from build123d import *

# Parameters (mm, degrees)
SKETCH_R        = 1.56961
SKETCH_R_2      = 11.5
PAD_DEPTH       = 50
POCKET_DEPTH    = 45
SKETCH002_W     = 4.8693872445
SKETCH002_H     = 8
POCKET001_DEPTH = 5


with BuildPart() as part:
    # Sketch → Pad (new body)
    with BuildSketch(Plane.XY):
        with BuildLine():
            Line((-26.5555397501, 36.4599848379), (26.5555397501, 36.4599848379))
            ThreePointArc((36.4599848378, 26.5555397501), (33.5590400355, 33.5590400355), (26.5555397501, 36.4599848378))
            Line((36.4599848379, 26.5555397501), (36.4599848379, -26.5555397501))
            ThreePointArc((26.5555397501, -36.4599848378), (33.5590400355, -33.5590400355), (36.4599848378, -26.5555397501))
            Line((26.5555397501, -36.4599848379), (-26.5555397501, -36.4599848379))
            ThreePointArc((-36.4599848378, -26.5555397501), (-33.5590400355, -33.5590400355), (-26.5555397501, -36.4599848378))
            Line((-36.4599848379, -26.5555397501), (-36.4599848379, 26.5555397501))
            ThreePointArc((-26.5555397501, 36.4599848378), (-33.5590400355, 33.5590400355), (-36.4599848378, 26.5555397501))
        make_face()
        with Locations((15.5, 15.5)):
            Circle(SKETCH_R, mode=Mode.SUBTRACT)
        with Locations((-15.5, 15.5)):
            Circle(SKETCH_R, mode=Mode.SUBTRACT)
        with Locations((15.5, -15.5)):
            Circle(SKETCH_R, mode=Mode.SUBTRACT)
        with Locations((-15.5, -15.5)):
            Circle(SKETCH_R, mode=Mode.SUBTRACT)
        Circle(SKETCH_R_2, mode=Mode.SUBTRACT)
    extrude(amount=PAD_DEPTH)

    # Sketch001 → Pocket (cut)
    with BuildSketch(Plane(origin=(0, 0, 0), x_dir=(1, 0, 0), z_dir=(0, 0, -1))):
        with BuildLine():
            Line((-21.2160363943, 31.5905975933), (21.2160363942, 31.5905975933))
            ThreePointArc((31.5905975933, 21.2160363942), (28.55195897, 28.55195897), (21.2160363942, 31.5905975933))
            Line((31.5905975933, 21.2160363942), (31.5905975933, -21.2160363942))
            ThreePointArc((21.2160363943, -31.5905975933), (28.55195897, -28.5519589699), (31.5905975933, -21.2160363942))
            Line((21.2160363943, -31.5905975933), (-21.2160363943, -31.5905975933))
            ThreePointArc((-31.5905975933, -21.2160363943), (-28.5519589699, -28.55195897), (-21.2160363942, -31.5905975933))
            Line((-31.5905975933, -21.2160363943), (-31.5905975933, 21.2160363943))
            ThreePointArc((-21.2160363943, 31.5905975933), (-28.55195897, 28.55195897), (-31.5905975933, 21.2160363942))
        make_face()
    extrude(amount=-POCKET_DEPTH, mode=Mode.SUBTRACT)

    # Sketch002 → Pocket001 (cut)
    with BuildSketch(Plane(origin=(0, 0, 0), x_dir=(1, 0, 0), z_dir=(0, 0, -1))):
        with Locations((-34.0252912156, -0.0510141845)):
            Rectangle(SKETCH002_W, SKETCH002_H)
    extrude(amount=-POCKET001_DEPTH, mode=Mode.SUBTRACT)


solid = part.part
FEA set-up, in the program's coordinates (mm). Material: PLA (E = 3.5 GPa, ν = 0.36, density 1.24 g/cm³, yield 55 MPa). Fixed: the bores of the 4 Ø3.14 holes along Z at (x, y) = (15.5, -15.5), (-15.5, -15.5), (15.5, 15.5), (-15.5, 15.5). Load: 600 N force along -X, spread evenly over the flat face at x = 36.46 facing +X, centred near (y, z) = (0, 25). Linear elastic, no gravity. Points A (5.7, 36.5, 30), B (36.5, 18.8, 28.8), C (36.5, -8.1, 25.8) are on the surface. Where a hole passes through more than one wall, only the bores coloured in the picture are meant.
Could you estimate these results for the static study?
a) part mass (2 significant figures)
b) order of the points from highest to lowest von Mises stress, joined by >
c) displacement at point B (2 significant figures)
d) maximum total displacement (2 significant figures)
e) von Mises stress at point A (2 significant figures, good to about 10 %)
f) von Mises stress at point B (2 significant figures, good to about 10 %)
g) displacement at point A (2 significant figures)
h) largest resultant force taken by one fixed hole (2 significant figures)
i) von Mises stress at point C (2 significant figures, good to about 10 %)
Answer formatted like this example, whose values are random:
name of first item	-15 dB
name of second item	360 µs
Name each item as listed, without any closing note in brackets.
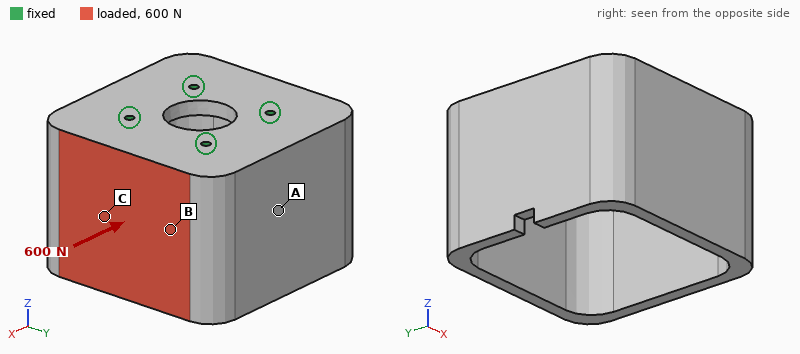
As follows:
part mass	100 g
order of the points from highest to lowest von Mises stress, joined by >	C > B > A
displacement at point B	0.32 mm
maximum total displacement	0.79 mm
von Mises stress at point A	2.2 MPa
von Mises stress at point B	4.7 MPa
displacement at point A	0.13 mm
largest resultant force taken by one fixed hole	300 N
von Mises stress at point C	6.2 MPa
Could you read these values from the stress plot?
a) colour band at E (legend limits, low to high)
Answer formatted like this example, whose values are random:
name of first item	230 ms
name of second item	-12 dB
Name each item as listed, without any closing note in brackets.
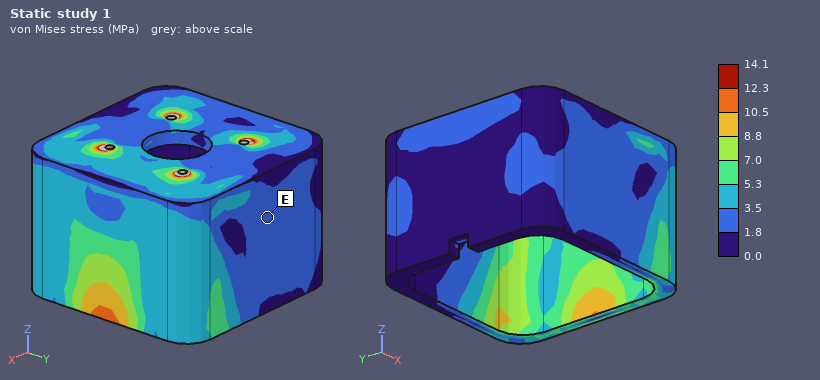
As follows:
colour band at E	1.8 to 3.5 MPa
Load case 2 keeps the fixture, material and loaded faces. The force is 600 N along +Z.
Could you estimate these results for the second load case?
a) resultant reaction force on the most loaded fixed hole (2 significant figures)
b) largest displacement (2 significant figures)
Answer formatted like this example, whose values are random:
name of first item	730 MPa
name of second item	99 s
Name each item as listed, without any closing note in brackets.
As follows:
resultant reaction force on the most loaded fixed hole	420 N
largest displacement	0.59 mm
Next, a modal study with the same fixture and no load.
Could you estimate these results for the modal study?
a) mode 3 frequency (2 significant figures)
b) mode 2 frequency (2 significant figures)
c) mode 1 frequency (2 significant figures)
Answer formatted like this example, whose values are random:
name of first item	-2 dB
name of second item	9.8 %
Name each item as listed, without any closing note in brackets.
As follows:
mode 3 frequency	820 Hz
mode 2 frequency	750 Hz
mode 1 frequency	750 Hz
